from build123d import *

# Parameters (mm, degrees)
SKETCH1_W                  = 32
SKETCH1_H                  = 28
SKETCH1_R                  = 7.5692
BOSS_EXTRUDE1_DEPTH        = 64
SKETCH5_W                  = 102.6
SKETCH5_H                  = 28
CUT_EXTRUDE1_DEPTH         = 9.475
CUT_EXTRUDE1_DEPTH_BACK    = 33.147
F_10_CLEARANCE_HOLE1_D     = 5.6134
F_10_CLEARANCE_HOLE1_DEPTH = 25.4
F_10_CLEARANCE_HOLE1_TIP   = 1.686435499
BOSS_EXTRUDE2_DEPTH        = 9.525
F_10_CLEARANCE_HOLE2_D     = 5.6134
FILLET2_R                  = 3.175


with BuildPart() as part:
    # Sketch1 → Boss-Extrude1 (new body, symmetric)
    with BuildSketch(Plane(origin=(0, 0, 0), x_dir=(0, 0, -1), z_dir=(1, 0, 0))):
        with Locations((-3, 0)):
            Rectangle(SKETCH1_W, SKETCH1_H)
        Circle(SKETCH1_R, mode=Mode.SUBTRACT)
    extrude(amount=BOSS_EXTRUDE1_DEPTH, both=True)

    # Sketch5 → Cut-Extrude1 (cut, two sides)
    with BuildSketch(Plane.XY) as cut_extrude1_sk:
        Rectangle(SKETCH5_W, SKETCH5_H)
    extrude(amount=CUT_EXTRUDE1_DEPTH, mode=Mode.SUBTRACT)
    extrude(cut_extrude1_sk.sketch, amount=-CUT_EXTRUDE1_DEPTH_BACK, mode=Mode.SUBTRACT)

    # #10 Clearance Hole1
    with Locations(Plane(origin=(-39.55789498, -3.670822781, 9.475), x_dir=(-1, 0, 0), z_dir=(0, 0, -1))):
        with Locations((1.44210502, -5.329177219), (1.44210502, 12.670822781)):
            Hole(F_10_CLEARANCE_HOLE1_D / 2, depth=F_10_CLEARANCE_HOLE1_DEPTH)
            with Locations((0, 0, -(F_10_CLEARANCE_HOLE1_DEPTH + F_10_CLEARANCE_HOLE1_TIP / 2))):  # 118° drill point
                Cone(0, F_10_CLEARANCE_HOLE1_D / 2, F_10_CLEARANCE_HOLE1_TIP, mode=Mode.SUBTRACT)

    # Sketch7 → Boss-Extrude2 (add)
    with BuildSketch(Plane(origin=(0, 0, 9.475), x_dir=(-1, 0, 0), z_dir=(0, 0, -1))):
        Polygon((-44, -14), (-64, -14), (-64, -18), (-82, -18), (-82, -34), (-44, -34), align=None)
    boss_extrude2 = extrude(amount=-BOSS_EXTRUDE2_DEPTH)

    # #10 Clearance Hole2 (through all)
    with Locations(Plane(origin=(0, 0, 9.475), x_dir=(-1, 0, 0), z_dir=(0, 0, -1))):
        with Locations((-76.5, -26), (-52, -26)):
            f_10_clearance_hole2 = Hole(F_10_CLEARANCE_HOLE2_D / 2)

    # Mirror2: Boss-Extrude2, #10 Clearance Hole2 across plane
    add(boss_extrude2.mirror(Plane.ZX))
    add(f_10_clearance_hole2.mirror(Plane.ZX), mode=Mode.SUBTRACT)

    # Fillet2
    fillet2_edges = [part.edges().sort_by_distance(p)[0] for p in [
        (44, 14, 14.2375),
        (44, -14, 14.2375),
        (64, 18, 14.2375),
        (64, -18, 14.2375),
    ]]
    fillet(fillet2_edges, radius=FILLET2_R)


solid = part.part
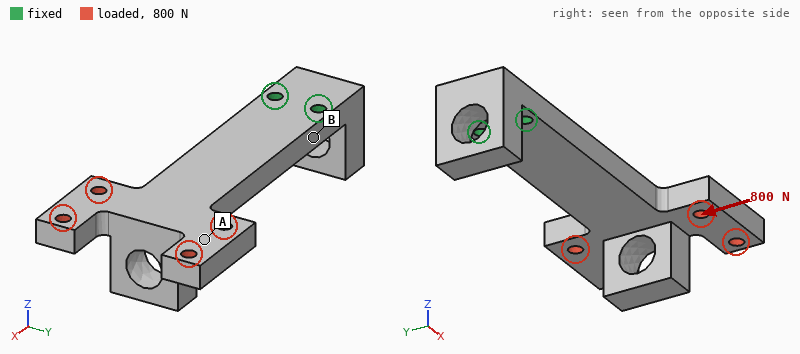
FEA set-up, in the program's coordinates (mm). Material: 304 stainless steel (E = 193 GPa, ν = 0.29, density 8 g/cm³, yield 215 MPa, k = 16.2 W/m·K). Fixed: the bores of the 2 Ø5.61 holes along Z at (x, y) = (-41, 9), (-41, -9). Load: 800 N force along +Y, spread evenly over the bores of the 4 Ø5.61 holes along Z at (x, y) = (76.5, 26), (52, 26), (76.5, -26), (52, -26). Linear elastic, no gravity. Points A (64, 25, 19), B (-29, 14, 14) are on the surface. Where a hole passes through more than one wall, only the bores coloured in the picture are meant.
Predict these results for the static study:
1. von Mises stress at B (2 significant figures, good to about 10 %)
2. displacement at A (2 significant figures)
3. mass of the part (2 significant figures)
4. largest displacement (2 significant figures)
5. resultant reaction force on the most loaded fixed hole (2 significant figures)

59 MPa
0.100 mm
460 g
0.13 mm
4.2 kN
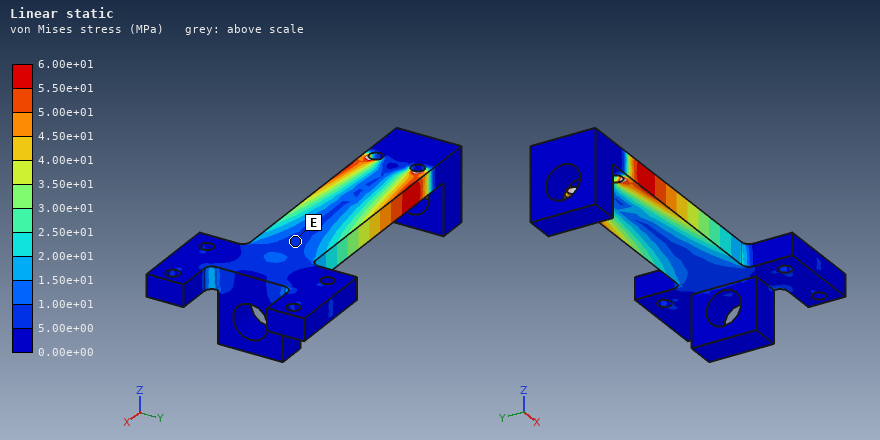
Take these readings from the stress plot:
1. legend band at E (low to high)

5.00e+00 to 1.00e+01 MPa
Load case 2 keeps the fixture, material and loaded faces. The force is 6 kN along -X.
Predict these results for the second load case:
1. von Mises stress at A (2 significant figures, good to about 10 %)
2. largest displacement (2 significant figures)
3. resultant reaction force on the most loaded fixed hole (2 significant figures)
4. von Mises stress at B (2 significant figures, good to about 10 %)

14 MPa
29 µm
3.0 kN
22 MPa
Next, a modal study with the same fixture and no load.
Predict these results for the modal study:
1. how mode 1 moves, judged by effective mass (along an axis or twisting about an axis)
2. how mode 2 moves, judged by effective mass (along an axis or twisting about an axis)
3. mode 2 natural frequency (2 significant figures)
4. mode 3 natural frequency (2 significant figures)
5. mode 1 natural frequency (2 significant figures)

along Z
along Y
1000 Hz
1300 Hz
370 Hz
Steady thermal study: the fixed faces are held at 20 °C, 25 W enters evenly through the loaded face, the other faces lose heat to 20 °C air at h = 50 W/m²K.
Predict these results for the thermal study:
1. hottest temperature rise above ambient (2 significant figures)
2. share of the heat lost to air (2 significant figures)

87 K
97 %
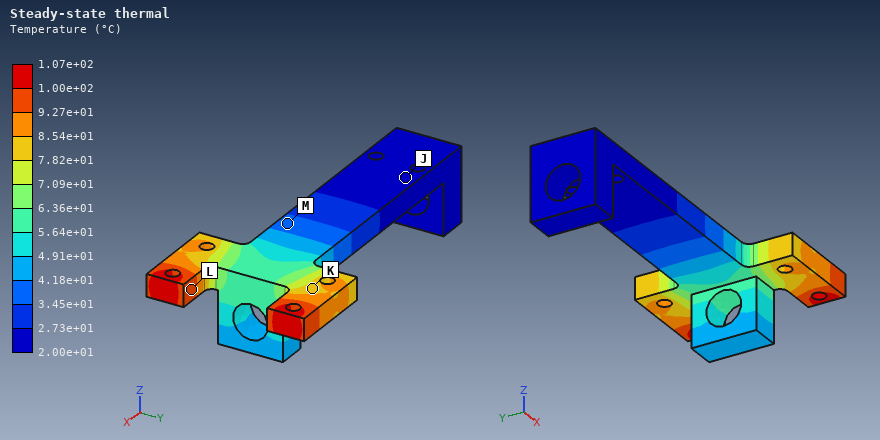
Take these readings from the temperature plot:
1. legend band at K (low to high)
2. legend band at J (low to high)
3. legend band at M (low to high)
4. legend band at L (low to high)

7.82e+01 to 8.54e+01 °C
2.00e+01 to 2.73e+01 °C
3.45e+01 to 4.18e+01 °C
9.27e+01 to 1.00e+02 °C
